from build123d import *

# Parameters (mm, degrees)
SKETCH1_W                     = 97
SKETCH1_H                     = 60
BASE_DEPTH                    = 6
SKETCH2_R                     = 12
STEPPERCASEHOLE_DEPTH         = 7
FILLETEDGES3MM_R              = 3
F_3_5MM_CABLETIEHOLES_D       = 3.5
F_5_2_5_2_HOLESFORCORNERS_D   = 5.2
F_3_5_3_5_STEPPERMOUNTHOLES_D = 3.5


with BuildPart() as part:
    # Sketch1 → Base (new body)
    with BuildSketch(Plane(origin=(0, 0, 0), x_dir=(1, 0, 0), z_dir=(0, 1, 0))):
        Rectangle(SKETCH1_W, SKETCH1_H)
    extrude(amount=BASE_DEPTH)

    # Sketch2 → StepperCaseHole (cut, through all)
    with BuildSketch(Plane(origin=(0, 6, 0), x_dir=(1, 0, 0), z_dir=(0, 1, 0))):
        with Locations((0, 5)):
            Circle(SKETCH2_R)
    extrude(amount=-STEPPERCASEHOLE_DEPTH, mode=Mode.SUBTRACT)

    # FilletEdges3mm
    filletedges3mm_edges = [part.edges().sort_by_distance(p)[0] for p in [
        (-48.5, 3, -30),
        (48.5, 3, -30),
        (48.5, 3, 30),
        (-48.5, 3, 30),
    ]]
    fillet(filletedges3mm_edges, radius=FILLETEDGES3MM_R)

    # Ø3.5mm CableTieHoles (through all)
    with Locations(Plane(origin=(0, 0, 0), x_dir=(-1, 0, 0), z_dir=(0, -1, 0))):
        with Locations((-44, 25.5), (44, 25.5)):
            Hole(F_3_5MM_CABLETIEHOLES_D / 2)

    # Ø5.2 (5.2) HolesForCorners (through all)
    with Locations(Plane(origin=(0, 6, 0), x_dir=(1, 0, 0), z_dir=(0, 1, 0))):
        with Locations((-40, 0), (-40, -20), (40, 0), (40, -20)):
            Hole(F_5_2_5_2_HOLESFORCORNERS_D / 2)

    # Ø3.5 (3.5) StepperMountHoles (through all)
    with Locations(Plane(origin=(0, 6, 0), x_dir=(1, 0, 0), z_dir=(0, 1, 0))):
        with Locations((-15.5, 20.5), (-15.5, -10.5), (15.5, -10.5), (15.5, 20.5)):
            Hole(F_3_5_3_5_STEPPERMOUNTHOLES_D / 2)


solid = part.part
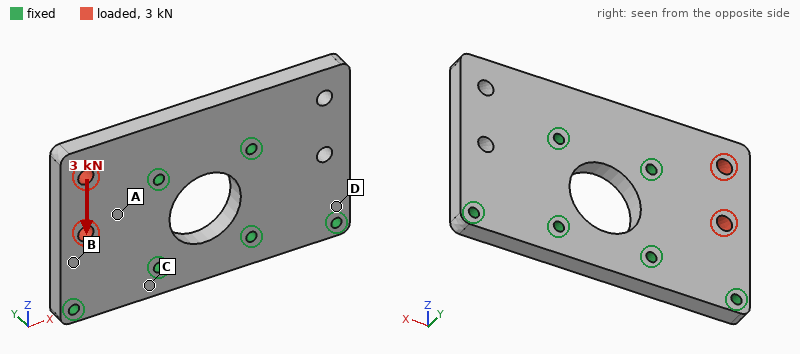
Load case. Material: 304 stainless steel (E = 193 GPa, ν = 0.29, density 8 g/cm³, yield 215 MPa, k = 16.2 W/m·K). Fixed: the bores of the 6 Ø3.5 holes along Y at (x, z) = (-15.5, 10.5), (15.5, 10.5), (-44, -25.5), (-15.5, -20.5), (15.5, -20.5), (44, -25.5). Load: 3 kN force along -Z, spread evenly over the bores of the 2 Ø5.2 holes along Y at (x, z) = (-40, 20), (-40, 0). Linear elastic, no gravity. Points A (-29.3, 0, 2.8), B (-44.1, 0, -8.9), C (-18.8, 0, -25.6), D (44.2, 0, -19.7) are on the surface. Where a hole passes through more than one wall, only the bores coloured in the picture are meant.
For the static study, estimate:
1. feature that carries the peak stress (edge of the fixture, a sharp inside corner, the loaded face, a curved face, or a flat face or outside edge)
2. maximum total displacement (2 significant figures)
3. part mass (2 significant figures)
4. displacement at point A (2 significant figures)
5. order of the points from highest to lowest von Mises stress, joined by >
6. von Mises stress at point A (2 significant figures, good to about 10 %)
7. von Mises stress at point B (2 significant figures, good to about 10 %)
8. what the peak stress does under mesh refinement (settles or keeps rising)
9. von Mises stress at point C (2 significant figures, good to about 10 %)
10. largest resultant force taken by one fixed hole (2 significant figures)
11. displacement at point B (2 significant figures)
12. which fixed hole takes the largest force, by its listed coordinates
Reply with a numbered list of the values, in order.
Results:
1. edge of the fixture
2. 5.1 µm
3. 250 g
4. 1.6 µm
5. B > A > C > D
6. 11 MPa
7. 22 MPa
8. keeps rising
9. 6.9 MPa
10. 1.4 kN
11. 1.9 µm
12. (-44, -25.5)
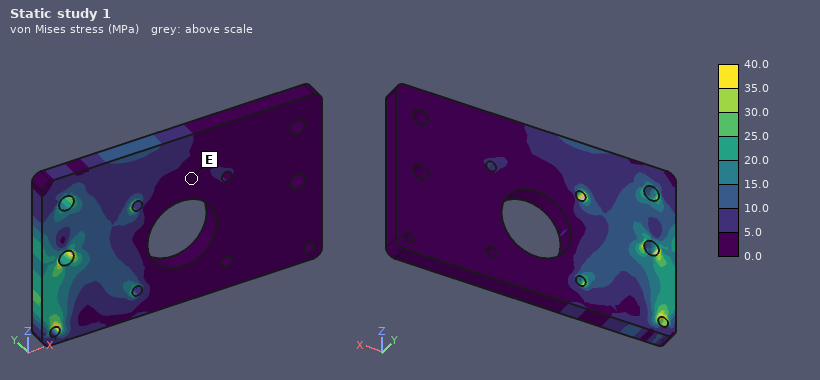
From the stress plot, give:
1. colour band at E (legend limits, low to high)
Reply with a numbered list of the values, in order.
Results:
1. 0.0 to 5.0 MPa
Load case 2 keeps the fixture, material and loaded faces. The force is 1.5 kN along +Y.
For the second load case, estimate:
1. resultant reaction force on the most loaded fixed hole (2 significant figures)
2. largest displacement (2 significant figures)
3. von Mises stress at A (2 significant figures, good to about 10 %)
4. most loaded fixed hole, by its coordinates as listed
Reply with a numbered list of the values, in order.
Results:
1. 1.4 kN
2. 78 µm
3. 51 MPa
4. (-15.5, 10.5)
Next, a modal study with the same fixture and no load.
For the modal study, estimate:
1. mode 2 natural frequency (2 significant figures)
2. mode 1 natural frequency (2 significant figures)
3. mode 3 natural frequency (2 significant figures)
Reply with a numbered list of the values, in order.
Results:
1. 4900 Hz
2. 4800 Hz
3. 9400 Hz
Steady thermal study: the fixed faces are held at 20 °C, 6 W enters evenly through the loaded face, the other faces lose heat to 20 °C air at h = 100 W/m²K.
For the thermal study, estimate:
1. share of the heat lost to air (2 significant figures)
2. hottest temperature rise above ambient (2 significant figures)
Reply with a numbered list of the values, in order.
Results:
1. 63 %
2. 22 K
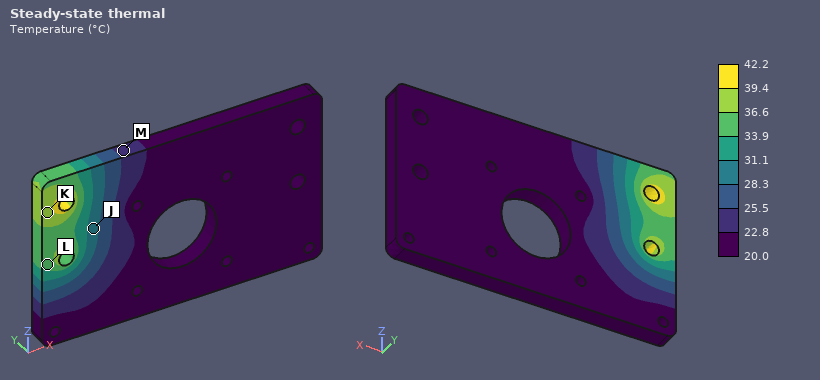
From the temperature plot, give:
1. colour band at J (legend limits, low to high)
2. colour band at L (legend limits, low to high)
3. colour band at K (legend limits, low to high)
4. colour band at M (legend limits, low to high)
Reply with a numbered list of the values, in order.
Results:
1. 28.3 to 31.1 °C
2. 33.9 to 36.6 °C
3. 36.6 to 39.4 °C
4. 22.8 to 25.5 °C
